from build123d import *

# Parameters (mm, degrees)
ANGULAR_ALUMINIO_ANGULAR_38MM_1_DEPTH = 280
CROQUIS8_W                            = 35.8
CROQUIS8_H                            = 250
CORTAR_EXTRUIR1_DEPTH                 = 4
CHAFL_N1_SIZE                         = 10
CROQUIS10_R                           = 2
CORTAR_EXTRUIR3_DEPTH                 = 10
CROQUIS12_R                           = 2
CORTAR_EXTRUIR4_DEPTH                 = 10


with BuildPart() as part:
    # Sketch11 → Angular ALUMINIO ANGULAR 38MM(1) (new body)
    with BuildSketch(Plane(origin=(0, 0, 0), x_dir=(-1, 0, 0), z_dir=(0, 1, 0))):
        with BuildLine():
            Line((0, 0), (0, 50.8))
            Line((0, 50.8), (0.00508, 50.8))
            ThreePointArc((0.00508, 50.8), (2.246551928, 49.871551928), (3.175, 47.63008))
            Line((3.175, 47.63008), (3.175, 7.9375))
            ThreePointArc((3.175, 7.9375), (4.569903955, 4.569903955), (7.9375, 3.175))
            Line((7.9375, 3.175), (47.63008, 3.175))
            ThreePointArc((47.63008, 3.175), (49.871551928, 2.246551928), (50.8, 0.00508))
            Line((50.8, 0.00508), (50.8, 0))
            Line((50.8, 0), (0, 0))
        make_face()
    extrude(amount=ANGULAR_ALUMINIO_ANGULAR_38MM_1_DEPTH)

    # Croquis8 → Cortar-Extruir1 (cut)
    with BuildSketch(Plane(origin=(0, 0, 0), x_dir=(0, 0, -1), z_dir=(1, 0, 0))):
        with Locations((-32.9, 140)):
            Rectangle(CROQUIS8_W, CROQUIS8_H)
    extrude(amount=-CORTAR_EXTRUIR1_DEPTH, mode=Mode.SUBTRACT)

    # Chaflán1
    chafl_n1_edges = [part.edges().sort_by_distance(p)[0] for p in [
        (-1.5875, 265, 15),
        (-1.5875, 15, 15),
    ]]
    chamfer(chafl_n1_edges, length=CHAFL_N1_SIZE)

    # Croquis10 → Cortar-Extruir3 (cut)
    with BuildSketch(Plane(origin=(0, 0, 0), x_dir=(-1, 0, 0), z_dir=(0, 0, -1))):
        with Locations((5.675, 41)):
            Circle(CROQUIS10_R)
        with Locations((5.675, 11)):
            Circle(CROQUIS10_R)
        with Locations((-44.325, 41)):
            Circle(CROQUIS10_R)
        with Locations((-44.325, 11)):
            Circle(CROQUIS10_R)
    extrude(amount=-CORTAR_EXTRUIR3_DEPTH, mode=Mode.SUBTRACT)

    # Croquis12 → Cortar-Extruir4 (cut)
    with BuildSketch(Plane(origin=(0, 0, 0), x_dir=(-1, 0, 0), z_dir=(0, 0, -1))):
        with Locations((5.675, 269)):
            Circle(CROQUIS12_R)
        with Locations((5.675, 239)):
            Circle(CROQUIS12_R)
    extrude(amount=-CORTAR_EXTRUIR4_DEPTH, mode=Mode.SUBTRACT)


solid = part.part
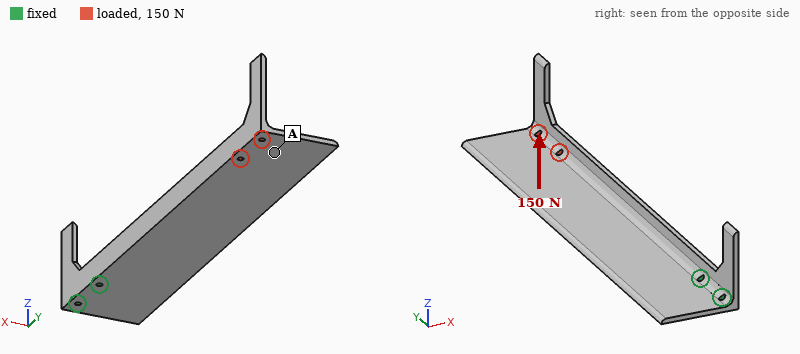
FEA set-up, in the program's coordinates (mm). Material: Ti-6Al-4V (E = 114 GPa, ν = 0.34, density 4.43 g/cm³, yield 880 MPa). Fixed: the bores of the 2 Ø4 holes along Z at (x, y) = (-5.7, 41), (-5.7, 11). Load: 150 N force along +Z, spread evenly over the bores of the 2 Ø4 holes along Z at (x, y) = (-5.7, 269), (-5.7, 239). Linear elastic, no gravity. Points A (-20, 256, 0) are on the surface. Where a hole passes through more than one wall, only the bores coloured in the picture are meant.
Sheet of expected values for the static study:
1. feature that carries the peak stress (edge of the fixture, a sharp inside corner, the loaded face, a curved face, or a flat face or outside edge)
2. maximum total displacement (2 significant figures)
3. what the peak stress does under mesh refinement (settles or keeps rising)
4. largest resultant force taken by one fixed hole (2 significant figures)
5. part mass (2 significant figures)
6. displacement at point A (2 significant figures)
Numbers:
edge of the fixture
3.4 mm
keeps rising
1.3 kN
270 g
2.9 mm
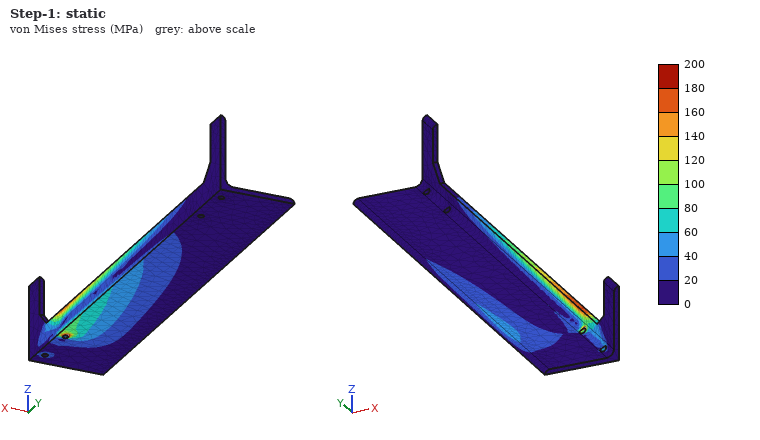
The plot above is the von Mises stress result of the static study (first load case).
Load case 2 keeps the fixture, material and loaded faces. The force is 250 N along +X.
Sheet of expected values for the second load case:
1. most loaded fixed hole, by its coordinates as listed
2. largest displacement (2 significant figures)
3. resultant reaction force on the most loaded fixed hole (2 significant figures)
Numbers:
(-5.7, 41)
0.71 mm
1.9 kN
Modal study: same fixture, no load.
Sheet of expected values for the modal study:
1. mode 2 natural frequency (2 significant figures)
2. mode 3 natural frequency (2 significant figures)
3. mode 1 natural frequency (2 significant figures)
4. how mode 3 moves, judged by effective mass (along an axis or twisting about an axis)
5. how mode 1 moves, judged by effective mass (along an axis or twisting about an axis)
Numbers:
310 Hz
530 Hz
120 Hz
along X
along Z
